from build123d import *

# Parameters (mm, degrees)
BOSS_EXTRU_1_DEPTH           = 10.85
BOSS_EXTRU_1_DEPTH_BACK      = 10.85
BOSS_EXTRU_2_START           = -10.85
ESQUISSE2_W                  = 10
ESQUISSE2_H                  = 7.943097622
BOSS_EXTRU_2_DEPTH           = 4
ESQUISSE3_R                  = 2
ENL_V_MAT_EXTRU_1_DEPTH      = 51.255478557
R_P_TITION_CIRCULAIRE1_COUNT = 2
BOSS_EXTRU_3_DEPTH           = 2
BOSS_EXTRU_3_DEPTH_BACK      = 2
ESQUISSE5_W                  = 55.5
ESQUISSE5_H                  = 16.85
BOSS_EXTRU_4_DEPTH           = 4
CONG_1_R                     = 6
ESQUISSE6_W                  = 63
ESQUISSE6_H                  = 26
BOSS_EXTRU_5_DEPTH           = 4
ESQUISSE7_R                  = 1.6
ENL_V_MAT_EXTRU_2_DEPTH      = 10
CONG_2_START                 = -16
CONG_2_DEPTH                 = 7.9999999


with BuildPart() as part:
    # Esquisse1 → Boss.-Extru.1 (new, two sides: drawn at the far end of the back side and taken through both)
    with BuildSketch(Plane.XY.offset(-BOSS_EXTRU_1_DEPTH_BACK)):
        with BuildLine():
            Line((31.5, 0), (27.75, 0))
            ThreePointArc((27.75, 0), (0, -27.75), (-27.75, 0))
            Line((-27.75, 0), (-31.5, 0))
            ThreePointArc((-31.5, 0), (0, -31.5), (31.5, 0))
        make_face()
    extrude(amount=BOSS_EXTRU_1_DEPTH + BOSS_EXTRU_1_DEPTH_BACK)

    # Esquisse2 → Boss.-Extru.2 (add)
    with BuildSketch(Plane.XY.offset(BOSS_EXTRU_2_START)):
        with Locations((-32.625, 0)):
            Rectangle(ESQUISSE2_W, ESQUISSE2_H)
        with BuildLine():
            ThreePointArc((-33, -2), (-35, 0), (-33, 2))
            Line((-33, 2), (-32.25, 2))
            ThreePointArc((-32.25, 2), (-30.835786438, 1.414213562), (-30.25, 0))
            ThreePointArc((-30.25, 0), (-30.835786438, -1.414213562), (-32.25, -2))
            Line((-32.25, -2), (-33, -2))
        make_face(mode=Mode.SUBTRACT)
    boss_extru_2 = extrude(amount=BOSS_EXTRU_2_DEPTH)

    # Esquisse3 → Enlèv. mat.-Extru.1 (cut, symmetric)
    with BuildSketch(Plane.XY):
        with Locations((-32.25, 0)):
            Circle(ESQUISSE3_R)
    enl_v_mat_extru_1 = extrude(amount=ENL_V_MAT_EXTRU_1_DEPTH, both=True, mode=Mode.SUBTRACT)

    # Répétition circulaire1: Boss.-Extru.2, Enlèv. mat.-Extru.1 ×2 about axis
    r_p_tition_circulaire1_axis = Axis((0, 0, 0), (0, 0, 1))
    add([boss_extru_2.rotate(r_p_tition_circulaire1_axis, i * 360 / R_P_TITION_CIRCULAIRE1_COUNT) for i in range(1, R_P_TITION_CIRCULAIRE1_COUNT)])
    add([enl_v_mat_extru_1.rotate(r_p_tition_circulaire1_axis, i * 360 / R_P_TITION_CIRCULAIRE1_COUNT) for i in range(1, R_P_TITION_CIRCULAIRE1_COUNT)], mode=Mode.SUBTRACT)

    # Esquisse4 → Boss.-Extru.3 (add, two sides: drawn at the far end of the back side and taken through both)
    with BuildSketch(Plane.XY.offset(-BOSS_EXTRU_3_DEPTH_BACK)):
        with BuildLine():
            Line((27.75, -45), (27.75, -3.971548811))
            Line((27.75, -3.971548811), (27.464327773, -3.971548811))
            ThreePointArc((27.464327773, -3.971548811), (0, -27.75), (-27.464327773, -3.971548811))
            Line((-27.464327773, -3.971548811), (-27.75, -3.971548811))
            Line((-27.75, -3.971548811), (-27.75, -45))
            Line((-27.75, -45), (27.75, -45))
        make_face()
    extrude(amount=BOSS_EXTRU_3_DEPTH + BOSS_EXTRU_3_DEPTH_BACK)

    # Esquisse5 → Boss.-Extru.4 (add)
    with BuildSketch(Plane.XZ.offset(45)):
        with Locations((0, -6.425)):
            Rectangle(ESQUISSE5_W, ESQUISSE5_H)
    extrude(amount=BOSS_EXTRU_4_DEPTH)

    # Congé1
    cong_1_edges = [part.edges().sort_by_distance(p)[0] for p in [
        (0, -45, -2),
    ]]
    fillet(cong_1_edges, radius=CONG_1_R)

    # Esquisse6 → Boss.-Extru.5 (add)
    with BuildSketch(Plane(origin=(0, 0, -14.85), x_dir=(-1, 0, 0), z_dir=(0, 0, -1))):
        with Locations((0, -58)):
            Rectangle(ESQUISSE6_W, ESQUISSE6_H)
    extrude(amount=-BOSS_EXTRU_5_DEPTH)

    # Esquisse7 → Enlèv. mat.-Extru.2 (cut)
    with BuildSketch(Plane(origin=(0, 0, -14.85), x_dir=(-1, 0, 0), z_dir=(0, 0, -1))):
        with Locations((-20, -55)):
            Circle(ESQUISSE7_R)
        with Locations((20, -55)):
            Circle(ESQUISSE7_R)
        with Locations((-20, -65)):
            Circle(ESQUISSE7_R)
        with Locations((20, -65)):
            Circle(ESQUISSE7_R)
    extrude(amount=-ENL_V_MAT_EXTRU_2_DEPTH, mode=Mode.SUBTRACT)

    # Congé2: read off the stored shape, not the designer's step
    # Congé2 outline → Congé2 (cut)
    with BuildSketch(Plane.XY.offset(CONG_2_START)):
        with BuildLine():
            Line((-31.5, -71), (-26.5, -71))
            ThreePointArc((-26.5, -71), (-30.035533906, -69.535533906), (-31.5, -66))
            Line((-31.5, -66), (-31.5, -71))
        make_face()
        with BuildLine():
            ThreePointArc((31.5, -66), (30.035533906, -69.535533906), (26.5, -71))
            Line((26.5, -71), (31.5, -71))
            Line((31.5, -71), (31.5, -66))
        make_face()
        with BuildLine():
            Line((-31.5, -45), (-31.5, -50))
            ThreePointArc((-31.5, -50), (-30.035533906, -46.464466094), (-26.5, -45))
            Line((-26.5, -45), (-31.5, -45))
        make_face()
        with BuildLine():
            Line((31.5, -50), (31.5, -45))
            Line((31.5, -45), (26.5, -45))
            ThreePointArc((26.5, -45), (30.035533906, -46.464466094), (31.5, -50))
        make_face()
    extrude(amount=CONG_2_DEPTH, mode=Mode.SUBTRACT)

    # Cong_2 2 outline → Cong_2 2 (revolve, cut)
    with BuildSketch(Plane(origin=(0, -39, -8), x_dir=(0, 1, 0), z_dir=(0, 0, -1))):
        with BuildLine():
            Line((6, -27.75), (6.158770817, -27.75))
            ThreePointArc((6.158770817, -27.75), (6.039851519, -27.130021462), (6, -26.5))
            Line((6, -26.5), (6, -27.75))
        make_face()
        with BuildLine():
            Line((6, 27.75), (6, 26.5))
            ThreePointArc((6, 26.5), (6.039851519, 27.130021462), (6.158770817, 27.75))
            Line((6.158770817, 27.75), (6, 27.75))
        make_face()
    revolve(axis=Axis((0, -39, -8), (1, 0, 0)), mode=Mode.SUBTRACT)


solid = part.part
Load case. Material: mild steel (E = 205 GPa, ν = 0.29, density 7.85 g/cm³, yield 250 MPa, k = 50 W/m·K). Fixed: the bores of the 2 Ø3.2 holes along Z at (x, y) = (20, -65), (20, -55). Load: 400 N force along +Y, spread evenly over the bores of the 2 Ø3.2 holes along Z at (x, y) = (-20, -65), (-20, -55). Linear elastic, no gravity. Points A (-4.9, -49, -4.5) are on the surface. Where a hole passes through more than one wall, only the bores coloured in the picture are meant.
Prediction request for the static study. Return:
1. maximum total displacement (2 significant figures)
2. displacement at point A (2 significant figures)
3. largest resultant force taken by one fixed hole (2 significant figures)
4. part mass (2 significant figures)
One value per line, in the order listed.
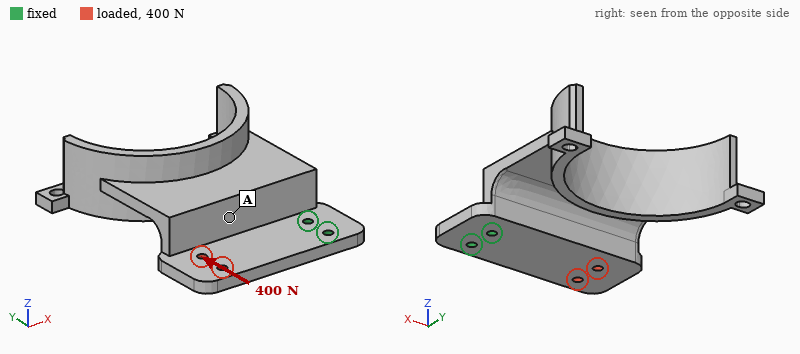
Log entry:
26 µm
7.6 µm
1.3 kN
170 g
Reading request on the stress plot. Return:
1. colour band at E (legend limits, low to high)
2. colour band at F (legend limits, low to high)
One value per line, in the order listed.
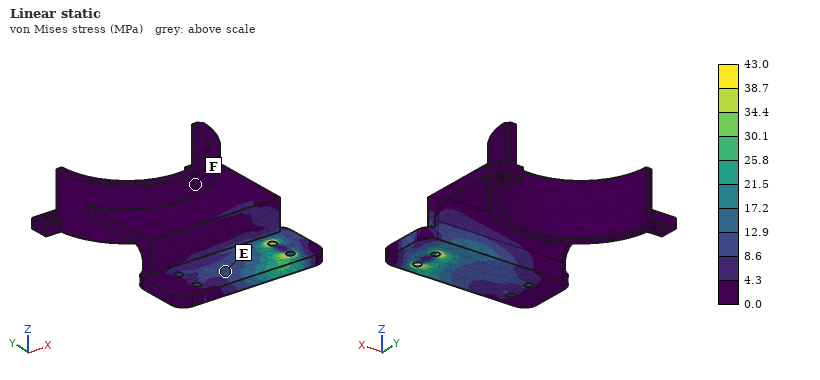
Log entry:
8.6 to 12.9 MPa
0.0 to 4.3 MPa
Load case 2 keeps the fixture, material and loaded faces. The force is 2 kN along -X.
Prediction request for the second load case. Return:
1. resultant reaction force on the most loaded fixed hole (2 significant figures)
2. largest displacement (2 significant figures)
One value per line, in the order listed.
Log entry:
1.0 kN
6.3 µm
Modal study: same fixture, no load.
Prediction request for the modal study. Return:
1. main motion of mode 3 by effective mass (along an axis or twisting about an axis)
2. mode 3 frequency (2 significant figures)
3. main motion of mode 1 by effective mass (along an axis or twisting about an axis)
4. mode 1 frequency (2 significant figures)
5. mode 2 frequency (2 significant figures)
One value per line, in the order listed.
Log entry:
along X
1700 Hz
along Z
650 Hz
1200 Hz
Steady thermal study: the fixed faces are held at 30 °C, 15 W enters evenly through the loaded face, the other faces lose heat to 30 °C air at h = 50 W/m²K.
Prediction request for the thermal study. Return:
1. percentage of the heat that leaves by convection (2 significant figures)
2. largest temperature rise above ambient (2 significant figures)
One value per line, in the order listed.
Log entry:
61 %
60 K
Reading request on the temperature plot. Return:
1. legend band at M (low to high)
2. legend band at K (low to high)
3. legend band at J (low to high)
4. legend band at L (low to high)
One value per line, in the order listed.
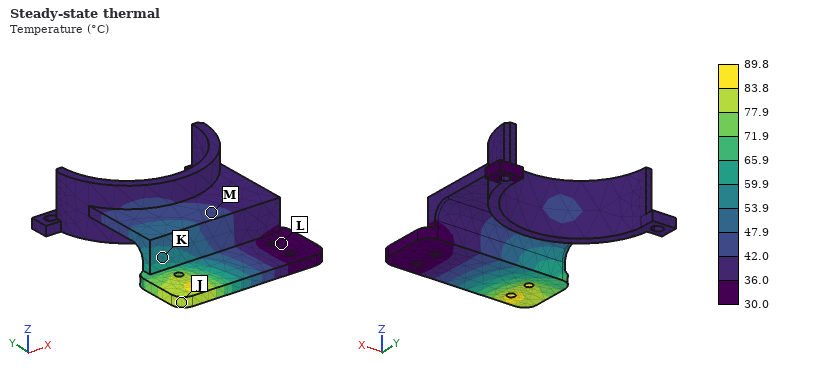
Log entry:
42.0 to 47.9 °C
53.9 to 59.9 °C
77.9 to 83.8 °C
30.0 to 36.0 °C
